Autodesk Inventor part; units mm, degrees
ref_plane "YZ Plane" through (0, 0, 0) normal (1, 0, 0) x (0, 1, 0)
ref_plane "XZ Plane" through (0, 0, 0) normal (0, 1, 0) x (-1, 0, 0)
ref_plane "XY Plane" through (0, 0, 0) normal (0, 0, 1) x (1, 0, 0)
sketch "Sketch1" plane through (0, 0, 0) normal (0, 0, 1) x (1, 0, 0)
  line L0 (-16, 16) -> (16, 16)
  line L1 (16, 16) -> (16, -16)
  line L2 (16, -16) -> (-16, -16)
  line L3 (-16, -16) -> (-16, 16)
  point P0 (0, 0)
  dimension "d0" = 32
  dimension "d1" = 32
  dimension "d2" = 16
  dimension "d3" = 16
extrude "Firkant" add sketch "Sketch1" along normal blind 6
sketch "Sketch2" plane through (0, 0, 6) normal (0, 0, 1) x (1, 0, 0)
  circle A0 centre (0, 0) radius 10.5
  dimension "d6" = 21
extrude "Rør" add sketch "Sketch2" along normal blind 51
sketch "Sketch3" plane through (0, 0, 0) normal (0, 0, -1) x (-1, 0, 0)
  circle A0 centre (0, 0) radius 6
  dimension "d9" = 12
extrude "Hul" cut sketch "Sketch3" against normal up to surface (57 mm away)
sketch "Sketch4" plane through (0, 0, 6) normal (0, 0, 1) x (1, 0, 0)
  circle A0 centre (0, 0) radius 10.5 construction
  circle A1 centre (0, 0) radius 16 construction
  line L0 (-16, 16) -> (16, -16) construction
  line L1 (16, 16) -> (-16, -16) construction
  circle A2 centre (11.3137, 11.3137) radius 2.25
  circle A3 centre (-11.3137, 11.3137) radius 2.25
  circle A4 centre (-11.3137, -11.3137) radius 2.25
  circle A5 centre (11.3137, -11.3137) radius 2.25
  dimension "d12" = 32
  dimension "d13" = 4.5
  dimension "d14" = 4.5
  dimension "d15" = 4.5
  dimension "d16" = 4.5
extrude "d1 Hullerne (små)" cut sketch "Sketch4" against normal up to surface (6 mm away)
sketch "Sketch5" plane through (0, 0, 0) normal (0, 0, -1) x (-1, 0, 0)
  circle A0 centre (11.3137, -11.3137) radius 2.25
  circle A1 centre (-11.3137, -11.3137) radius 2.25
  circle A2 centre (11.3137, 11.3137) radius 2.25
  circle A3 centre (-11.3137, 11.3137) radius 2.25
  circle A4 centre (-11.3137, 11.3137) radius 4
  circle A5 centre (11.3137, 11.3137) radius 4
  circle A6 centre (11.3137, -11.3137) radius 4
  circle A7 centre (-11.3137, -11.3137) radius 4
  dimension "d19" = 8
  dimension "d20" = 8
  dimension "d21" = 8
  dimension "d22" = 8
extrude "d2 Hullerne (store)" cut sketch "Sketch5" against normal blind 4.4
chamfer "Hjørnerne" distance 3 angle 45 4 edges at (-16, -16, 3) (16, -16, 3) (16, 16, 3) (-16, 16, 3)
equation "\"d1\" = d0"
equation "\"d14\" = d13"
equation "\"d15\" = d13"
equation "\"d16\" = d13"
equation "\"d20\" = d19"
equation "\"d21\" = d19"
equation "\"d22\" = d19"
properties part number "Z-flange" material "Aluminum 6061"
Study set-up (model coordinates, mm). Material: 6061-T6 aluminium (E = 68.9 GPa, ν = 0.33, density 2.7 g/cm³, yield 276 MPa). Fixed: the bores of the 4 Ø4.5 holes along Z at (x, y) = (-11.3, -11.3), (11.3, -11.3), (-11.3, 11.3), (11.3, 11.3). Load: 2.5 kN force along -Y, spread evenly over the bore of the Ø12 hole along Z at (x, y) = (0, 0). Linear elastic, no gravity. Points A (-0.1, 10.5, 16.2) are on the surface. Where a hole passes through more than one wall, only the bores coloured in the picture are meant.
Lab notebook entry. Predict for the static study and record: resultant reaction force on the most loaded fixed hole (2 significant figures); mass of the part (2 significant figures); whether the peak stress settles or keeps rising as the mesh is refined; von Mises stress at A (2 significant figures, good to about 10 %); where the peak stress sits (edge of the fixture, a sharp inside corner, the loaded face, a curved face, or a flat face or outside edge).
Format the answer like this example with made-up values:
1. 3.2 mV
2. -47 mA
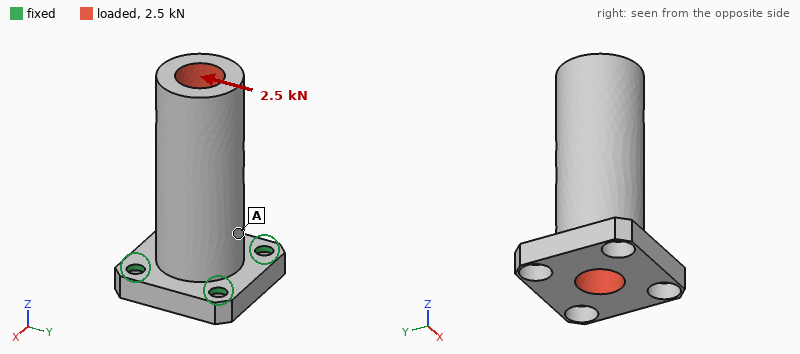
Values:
1. 1.5 kN
2. 44 g
3. keeps rising
4. 42 MPa
5. edge of the fixture
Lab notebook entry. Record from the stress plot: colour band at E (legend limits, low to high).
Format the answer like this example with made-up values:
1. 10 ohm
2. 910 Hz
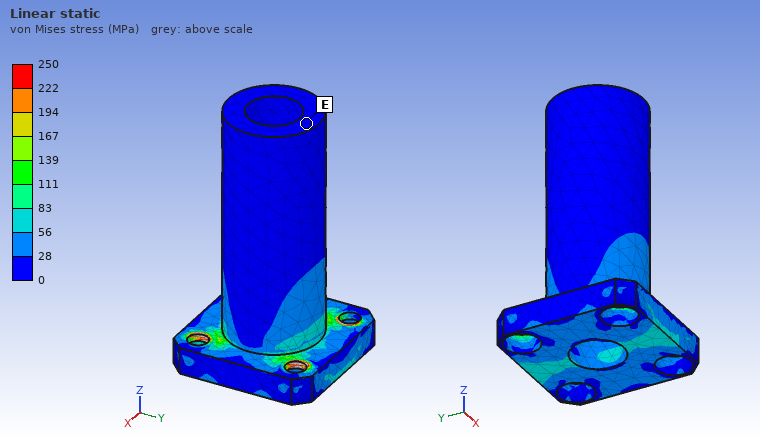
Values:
1. 0 to 28 MPa
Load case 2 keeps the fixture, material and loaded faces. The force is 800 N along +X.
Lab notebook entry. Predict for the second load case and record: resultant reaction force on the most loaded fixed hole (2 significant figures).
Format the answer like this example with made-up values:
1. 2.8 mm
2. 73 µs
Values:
1. 480 N
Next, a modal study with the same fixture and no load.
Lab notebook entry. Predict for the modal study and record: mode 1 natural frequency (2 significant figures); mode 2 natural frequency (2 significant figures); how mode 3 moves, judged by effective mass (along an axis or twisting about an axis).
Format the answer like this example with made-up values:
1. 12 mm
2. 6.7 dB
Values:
1. 3600 Hz
2. 3600 Hz
3. along Z
